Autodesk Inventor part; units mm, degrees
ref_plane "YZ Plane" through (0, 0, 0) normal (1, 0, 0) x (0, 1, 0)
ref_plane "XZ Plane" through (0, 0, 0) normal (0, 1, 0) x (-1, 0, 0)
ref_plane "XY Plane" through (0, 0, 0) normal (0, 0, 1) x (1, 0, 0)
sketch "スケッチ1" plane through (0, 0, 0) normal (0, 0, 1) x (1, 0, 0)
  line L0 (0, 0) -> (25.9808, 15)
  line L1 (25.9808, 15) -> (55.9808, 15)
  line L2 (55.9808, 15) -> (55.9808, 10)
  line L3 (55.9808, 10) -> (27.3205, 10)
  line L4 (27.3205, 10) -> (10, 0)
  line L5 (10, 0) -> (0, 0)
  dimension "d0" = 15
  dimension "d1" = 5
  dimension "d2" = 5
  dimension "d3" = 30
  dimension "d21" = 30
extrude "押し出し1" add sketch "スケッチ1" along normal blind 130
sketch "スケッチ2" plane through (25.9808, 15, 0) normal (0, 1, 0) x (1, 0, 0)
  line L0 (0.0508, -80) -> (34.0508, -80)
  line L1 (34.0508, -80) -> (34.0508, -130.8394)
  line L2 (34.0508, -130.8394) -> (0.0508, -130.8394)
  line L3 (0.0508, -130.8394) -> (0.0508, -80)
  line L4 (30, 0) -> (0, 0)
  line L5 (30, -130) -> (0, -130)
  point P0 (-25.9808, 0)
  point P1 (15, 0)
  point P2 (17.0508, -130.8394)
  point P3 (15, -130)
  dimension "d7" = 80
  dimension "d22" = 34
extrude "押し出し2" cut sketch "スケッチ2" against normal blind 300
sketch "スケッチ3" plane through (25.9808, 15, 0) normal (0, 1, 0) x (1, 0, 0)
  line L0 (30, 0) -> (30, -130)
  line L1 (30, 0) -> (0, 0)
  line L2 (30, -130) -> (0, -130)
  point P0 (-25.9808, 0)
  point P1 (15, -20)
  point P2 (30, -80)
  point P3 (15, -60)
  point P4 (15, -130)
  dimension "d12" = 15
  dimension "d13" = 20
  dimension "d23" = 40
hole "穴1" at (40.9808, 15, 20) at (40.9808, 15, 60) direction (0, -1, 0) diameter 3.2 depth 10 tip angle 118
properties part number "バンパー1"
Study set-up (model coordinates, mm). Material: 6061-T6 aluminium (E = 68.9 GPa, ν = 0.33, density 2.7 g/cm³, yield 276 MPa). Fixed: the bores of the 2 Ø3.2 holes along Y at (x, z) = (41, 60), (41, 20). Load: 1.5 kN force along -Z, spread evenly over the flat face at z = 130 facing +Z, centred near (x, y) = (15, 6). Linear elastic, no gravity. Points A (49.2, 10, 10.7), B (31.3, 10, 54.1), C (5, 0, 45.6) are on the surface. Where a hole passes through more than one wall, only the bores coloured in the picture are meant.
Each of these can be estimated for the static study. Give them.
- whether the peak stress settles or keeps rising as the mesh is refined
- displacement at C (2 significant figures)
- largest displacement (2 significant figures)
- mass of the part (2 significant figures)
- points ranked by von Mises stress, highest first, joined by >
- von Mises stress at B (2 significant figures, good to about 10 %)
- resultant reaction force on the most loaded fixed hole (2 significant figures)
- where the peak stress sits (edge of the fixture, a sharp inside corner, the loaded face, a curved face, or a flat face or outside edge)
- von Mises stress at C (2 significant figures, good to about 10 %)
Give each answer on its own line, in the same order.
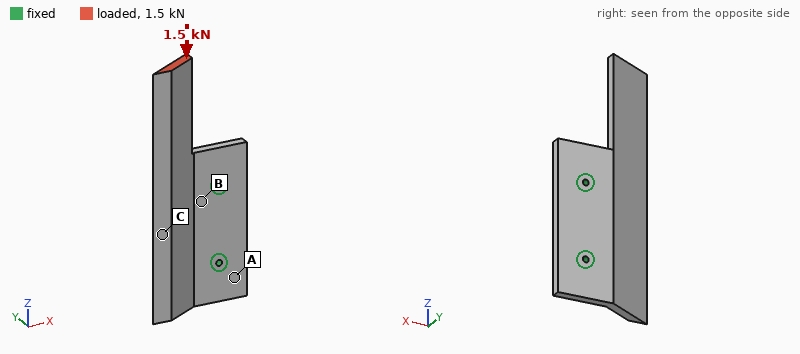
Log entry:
keeps rising
16 µm
78 µm
75 g
B > C > A
20 MPa
1.2 kN
edge of the fixture
11 MPa
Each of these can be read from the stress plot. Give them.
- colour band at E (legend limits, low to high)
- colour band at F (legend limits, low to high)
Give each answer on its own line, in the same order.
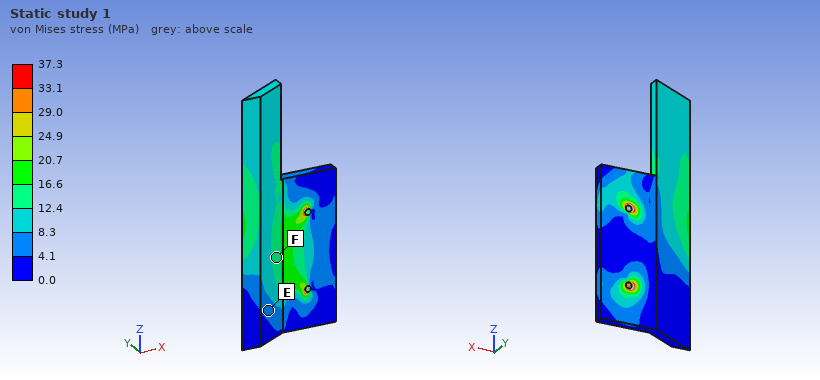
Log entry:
4.1 to 8.3 MPa
12.4 to 16.6 MPa
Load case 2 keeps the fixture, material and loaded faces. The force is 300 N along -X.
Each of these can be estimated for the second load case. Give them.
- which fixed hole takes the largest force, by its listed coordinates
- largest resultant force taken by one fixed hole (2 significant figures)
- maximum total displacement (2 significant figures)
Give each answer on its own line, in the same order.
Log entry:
(41, 60)
820 N
0.85 mm
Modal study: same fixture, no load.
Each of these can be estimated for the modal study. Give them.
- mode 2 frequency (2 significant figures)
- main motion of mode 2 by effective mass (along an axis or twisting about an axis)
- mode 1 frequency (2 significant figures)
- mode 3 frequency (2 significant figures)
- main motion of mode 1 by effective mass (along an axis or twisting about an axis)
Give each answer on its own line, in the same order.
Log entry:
2100 Hz
along Y
810 Hz
2800 Hz
along Y
